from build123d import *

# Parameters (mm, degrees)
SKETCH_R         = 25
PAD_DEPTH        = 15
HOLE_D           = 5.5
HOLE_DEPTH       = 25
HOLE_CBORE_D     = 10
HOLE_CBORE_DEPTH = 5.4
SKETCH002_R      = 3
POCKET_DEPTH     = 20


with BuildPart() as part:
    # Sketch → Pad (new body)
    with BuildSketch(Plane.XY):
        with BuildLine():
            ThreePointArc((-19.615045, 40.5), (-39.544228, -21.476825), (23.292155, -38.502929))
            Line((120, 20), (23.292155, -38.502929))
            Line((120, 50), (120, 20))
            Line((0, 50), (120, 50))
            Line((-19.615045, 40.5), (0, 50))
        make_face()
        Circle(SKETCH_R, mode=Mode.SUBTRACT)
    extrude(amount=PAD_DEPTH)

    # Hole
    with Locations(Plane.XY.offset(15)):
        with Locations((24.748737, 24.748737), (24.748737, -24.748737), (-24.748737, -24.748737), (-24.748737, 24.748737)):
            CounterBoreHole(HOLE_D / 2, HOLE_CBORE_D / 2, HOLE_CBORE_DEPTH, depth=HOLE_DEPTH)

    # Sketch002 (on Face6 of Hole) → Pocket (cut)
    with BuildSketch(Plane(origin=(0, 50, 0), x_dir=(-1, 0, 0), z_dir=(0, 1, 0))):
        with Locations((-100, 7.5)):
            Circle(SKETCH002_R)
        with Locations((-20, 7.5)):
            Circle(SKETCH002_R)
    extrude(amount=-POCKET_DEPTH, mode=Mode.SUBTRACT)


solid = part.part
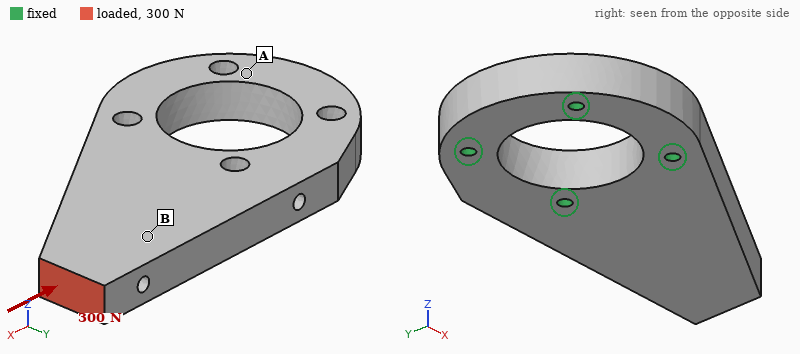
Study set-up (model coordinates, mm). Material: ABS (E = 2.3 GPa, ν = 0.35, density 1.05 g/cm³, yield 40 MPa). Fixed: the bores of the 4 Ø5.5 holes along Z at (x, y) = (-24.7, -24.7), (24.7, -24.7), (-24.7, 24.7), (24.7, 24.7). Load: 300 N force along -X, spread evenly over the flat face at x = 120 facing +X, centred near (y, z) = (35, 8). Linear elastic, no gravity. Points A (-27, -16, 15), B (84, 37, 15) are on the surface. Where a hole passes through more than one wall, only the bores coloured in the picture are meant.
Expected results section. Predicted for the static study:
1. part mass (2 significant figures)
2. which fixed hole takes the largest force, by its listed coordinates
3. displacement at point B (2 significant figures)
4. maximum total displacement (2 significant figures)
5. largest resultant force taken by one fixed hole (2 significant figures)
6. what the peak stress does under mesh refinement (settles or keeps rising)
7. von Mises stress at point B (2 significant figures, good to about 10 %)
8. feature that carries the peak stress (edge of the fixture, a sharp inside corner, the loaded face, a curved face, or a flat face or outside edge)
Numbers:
140 g
(24.7, 24.7)
35 µm
69 µm
250 N
keeps rising
0.64 MPa
edge of the fixture
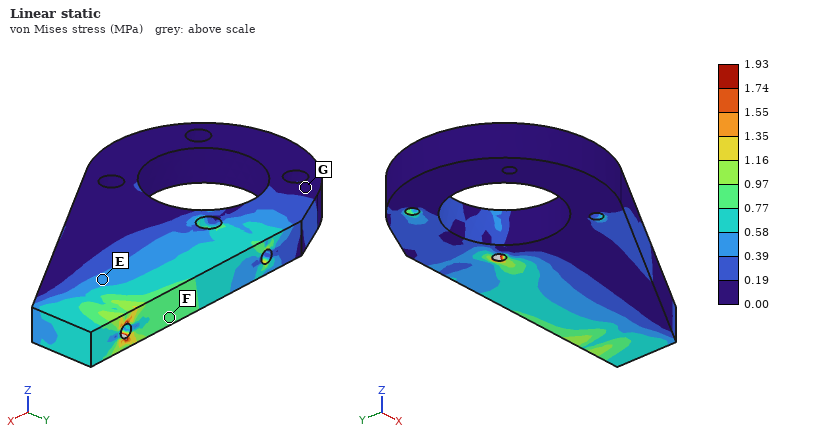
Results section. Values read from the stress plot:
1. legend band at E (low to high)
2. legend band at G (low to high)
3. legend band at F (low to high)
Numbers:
0.39 to 0.58 MPa
0.00 to 0.19 MPa
0.77 to 0.97 MPa
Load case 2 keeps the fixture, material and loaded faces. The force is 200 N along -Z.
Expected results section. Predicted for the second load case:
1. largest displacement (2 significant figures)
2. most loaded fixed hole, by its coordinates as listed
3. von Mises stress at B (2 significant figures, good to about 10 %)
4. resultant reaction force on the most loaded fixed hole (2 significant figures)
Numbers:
2.2 mm
(24.7, 24.7)
4.0 MPa
420 N
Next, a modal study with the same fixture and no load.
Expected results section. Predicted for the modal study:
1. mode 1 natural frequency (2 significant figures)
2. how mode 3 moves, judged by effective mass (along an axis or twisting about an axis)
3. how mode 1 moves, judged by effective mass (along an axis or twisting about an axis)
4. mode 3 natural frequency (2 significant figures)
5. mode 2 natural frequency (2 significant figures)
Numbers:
380 Hz
along Y
along Z
1500 Hz
1500 Hz
